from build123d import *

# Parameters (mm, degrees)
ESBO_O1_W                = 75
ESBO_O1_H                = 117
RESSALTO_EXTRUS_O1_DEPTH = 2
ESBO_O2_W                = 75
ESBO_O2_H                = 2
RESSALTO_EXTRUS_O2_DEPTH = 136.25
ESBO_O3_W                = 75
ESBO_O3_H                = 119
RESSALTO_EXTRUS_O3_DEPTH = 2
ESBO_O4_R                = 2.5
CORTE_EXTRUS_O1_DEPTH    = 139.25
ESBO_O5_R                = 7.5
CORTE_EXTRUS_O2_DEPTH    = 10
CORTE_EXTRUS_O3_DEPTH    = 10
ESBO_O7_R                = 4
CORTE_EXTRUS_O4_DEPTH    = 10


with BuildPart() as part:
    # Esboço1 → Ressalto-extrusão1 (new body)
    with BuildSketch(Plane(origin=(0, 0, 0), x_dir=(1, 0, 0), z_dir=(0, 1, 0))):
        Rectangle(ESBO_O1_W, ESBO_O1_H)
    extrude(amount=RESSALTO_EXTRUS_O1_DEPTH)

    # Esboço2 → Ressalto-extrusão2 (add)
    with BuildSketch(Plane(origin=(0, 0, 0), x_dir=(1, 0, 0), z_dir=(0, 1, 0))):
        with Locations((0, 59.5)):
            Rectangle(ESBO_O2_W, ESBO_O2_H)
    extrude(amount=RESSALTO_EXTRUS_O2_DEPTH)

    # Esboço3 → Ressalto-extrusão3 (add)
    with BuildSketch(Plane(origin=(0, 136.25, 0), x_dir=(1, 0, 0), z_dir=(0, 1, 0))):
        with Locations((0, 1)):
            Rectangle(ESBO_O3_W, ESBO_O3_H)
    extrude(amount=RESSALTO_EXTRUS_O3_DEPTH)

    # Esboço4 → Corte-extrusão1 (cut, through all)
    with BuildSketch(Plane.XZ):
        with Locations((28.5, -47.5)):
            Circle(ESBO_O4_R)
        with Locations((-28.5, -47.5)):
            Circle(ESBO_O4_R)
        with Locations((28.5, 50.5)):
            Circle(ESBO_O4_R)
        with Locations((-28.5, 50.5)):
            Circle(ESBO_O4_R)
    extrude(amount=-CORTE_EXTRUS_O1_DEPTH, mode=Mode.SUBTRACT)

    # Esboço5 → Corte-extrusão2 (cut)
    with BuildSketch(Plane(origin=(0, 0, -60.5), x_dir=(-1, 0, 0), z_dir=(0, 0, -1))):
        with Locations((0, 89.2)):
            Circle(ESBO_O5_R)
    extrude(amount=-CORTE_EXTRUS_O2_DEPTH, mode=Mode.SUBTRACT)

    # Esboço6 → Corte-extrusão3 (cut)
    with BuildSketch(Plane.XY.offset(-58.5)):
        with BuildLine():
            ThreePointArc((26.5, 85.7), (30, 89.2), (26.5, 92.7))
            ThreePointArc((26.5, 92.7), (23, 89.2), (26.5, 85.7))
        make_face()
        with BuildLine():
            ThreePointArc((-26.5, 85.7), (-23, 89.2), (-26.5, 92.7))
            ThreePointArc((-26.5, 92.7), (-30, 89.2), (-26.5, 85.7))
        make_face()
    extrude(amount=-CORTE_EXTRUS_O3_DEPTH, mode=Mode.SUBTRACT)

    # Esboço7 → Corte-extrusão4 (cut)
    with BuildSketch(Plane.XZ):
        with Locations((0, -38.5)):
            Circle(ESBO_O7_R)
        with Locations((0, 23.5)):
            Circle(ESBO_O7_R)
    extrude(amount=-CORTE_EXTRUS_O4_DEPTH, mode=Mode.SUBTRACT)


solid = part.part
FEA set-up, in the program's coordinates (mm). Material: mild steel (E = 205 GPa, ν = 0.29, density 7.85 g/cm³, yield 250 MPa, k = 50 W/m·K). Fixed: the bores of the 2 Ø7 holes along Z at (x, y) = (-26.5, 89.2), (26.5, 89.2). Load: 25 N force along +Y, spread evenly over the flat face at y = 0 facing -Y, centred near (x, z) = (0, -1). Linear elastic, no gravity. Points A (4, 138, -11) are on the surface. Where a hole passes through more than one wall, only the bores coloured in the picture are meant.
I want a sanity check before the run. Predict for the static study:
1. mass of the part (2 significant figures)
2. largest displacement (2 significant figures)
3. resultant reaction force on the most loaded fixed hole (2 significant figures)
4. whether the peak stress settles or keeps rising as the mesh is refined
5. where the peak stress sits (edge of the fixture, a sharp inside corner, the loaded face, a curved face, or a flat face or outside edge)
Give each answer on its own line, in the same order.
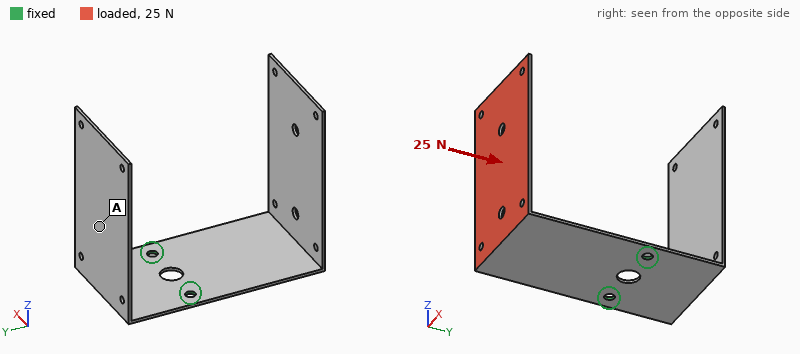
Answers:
430 g
2.0 mm
13 N
keeps rising
edge of the fixture
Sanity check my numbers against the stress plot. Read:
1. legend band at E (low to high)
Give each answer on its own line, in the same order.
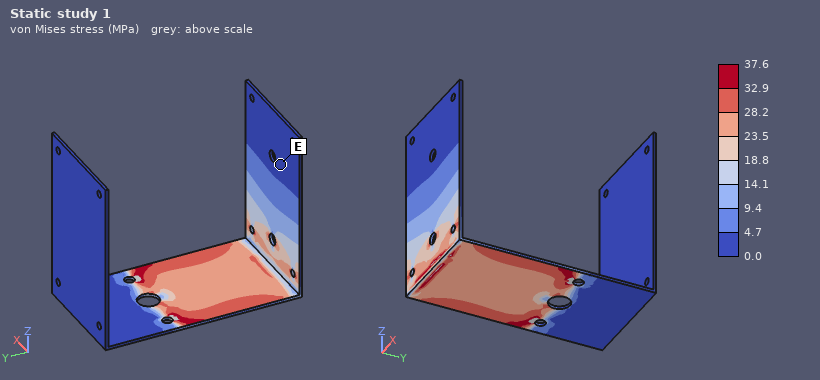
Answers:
0.0 to 4.7 MPa
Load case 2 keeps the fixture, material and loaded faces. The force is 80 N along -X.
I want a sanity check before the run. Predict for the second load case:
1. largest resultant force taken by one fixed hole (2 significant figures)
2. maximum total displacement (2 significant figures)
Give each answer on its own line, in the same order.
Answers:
160 N
2.2 mm
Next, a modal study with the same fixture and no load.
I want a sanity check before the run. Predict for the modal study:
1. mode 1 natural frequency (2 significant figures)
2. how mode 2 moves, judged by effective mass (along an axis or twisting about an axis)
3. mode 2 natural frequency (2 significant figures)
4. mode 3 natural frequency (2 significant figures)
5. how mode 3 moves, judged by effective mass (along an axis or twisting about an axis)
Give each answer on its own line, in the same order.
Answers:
52 Hz
along Y
73 Hz
97 Hz
along X
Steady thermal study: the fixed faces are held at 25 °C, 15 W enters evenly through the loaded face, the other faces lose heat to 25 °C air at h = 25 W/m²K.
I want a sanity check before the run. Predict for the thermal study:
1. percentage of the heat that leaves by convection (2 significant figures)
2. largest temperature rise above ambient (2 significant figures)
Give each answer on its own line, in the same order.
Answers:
93 %
52 K
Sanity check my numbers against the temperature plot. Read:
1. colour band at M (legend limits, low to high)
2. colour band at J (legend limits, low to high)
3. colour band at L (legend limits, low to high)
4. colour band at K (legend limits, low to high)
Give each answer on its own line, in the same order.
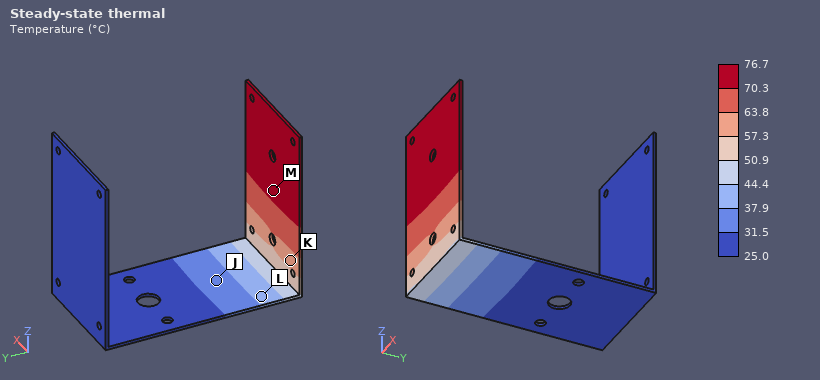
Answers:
70.3 to 76.7 °C
31.5 to 37.9 °C
37.9 to 44.4 °C
57.3 to 63.8 °C
